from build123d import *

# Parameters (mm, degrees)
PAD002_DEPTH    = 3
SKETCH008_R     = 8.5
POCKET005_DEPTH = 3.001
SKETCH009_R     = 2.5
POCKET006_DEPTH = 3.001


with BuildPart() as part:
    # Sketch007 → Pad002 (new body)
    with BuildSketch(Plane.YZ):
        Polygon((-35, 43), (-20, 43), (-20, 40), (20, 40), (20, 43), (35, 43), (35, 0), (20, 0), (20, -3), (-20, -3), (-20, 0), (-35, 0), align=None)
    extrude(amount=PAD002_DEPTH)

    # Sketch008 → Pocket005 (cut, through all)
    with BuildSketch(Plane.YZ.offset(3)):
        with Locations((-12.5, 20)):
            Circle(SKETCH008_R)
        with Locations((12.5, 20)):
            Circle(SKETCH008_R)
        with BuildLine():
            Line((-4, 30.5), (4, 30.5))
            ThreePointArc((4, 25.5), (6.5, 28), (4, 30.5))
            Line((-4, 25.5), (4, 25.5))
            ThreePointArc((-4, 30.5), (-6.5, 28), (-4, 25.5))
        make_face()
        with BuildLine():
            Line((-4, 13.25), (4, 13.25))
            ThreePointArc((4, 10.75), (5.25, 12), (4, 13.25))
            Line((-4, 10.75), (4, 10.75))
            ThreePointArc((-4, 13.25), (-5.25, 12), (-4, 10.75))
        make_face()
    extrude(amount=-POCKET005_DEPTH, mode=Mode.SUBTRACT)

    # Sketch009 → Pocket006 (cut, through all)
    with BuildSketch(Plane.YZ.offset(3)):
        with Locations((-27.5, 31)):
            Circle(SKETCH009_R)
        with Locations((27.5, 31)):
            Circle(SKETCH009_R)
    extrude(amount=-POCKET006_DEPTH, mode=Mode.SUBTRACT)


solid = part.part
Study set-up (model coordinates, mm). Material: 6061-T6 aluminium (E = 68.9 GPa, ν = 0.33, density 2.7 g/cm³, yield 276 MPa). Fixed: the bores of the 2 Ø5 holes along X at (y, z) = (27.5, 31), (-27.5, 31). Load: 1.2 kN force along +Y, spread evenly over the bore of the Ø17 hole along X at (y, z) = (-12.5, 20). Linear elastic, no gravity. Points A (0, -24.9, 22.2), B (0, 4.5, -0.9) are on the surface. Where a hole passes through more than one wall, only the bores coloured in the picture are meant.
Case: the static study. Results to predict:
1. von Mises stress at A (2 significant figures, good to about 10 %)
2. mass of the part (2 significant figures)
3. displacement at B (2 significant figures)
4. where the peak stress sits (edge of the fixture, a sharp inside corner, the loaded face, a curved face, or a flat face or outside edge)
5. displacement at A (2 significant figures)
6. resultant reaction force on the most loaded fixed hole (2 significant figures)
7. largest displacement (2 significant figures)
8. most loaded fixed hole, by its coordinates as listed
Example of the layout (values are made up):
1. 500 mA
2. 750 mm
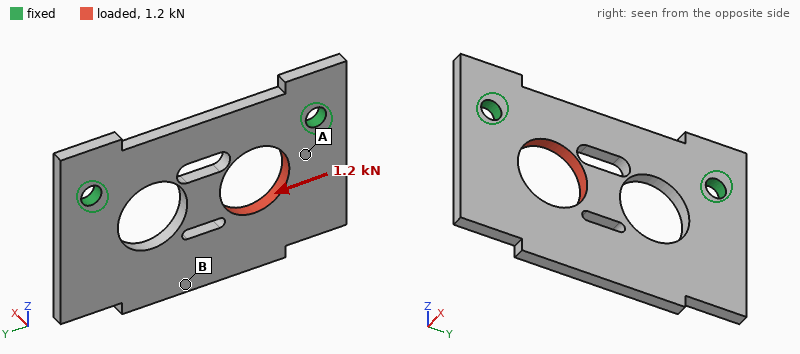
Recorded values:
1. 18 MPa
2. 20 g
3. 12 µm
4. a curved face
5. 5.6 µm
6. 850 N
7. 16 µm
8. (-27.5, 31)
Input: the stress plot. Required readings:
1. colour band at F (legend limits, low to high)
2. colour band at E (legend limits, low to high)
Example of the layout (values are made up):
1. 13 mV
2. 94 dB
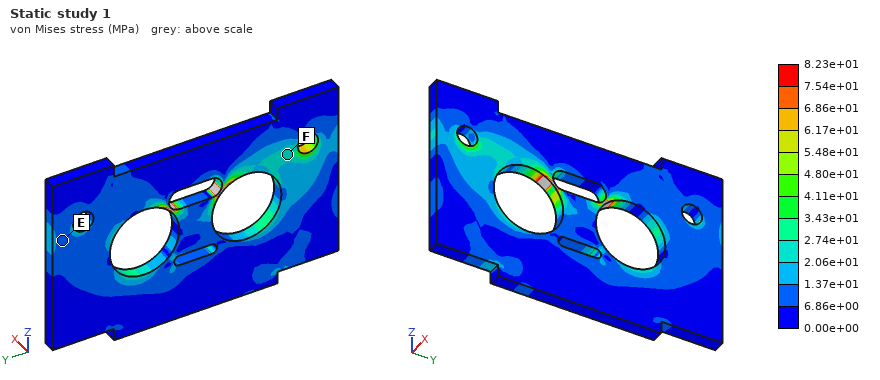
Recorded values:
1. 2.06e+01 to 2.74e+01 MPa
2. 6.86e+00 to 1.37e+01 MPa
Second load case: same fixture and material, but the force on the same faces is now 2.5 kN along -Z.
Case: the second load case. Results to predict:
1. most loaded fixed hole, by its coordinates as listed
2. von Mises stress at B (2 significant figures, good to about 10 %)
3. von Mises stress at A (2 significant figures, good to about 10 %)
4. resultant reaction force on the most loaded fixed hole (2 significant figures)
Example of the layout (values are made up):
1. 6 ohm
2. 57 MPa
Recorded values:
1. (-27.5, 31)
2. 20 MPa
3. 51 MPa
4. 1.9 kN
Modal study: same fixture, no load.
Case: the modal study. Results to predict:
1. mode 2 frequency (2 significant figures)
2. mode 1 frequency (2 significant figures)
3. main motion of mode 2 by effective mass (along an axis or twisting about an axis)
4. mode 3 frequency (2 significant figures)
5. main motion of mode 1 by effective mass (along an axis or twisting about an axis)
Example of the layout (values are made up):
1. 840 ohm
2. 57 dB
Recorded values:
1. 3300 Hz
2. 1600 Hz
3. twisting about Z
4. 5100 Hz
5. along X
